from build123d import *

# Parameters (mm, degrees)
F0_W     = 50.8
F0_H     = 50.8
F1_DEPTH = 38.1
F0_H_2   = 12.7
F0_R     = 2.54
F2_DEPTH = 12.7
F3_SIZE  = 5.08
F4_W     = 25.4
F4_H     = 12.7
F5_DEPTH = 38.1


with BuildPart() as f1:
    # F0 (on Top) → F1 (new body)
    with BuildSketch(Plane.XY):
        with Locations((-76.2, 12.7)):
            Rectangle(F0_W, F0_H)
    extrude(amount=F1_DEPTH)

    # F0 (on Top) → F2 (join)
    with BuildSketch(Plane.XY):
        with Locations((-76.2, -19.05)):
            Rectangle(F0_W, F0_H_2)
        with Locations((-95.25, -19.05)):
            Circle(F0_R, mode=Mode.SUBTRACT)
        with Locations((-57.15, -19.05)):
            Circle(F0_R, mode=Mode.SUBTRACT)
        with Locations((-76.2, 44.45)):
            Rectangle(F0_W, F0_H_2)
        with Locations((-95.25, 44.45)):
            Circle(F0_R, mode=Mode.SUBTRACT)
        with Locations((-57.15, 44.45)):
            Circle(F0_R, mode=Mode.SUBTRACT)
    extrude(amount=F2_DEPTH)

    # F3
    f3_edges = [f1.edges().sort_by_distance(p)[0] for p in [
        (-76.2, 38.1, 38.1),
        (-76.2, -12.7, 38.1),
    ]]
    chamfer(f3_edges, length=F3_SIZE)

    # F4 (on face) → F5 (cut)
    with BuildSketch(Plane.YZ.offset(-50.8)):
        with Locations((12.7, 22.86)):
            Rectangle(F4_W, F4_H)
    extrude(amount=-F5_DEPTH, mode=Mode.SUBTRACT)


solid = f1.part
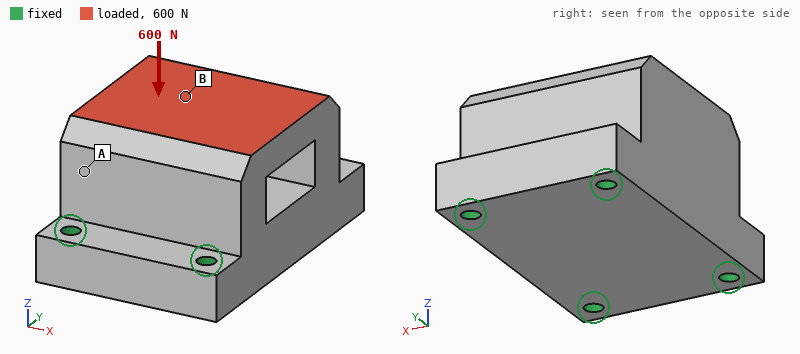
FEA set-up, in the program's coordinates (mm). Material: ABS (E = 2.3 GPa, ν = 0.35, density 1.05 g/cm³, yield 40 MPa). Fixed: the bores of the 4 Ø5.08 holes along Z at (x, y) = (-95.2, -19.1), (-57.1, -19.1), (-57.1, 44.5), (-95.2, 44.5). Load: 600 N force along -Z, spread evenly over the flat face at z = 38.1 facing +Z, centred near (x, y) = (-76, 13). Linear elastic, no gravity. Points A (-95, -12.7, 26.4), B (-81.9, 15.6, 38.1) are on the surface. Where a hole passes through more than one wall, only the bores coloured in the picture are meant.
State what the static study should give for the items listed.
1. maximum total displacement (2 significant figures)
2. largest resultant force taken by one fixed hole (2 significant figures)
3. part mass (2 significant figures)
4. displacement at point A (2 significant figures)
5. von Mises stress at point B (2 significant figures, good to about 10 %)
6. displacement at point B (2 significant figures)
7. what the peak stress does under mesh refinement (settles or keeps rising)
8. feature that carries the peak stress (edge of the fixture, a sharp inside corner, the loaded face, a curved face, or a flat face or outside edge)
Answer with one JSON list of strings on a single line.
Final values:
["30 µm", "160 N", "110 g", "13 µm", "0.59 MPa", "22 µm", "keeps rising", "edge of the fixture"]
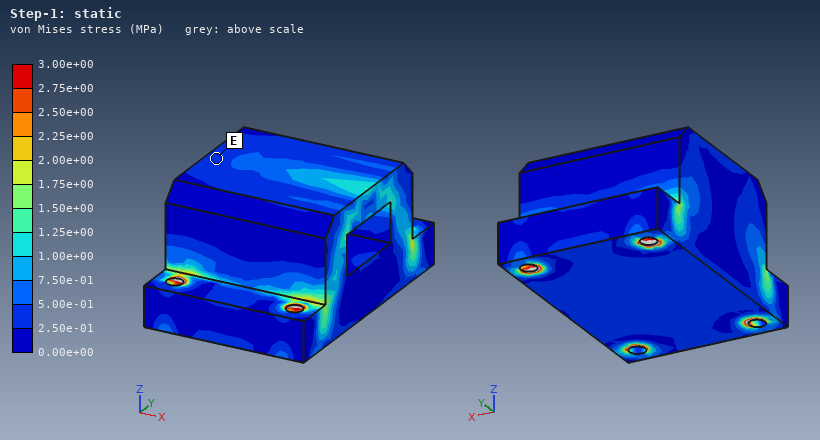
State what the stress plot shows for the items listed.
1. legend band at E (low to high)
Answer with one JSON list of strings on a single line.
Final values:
["2.50e-01 to 5.00e-01 MPa"]
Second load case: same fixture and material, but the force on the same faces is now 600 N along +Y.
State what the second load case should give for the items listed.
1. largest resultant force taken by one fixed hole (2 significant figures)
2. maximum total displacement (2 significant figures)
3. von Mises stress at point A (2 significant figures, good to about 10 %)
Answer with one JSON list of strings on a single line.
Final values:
["250 N", "50 µm", "0.52 MPa"]
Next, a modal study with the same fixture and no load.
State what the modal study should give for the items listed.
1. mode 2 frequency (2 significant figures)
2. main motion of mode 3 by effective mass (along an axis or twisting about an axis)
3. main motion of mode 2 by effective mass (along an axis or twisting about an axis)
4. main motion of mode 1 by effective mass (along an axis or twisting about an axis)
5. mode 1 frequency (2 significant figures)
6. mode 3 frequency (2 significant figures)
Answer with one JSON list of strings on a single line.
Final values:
["3400 Hz", "along Y", "along Z", "along X", "2700 Hz", "3600 Hz"]
